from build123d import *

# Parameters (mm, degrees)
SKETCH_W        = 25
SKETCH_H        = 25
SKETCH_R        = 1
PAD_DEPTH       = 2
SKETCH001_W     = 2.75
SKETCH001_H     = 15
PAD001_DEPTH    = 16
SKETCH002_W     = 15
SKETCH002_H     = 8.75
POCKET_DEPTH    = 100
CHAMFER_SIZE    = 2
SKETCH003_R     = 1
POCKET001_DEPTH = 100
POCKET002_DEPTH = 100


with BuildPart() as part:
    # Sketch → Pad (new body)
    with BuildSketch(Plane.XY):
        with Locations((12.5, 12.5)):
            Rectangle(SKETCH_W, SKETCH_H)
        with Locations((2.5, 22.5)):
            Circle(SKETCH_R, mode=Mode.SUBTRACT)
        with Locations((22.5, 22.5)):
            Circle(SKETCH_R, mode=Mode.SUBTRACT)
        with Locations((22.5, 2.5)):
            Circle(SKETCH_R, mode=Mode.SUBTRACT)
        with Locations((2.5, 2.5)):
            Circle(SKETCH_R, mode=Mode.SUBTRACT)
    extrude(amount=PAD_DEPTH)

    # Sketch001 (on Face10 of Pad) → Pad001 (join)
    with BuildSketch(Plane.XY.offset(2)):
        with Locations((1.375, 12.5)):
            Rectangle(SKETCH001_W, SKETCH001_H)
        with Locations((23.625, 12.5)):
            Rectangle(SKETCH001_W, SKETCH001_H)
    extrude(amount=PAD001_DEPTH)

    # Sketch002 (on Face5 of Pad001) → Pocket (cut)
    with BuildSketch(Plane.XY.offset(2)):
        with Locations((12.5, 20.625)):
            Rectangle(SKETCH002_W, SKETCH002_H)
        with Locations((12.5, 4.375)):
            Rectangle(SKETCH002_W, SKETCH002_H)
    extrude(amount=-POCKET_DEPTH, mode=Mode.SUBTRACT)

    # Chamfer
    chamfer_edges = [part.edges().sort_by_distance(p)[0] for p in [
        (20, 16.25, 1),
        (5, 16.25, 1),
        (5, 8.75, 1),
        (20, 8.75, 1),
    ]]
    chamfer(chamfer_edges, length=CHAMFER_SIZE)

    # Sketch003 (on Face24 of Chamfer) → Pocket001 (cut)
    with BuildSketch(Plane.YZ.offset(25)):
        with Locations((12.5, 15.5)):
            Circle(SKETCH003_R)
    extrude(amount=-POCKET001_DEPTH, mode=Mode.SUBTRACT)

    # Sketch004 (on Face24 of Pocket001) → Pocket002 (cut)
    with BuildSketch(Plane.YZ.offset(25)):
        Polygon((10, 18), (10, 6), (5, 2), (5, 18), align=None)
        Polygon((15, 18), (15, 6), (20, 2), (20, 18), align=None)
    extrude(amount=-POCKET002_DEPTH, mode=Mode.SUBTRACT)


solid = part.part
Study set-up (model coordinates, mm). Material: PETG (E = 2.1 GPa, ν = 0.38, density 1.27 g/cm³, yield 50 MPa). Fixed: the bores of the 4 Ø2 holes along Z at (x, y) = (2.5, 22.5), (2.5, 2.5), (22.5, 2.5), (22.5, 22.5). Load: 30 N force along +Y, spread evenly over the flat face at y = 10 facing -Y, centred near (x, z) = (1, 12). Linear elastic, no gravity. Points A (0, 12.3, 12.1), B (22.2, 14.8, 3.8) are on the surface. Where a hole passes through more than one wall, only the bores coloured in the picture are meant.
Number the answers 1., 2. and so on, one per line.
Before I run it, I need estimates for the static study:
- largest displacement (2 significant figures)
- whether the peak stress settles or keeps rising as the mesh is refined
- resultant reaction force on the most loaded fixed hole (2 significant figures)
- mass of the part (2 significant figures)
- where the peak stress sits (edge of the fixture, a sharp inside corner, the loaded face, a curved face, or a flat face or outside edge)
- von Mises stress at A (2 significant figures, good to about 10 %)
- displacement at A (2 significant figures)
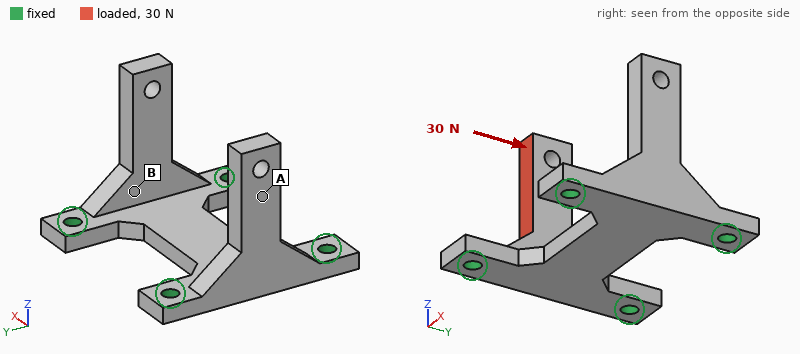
1. 0.30 mm
2. keeps rising
3. 25 N
4. 1.6 g
5. edge of the fixture
6. 3.1 MPa
7. 0.15 mm
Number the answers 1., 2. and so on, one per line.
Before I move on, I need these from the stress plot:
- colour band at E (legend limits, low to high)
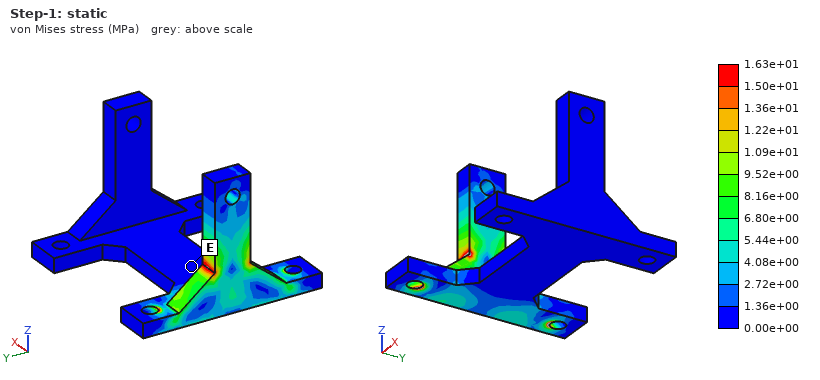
1. 0.00e+00 to 1.36e+00 MPa
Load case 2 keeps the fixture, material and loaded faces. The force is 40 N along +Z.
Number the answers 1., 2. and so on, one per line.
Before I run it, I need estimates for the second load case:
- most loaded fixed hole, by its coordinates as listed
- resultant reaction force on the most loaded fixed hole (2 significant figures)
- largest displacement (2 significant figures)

1. (2.5, 2.5)
2. 31 N
3. 0.22 mm
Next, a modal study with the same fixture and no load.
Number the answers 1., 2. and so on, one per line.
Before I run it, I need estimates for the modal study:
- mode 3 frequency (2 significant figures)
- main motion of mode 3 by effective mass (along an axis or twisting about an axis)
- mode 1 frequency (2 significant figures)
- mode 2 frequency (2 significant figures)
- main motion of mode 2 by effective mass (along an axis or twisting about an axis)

1. 4400 Hz
2. along Y
3. 1600 Hz
4. 1800 Hz
5. along X
